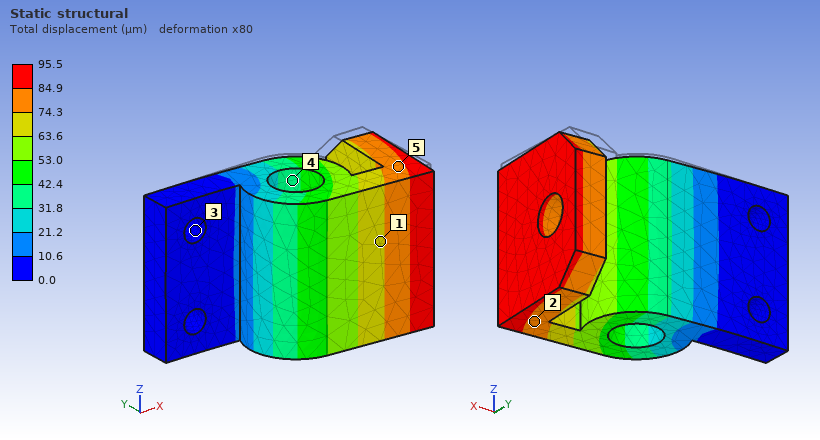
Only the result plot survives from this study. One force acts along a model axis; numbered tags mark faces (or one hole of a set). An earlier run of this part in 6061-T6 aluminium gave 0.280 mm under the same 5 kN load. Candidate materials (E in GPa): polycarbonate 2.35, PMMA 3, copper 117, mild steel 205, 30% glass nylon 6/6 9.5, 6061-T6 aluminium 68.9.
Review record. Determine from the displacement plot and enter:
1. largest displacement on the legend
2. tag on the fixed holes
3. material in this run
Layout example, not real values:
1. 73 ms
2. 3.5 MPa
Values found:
1. 95.5 µm
2. 3
3. mild steel
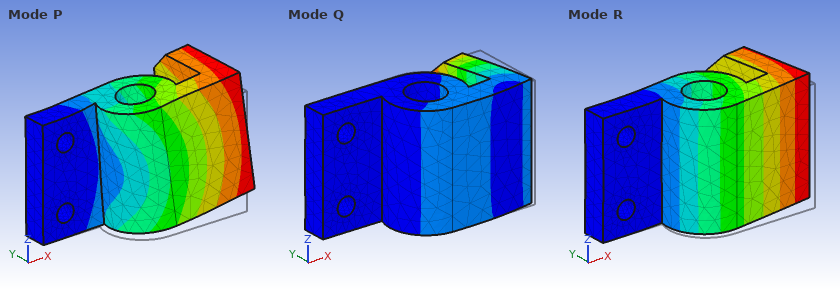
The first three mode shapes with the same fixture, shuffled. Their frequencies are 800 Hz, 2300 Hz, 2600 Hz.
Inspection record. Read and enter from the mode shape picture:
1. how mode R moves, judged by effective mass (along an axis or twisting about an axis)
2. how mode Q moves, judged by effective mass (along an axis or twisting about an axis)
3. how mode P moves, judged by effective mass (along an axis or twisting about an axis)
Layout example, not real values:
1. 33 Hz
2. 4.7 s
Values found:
1. along Y
2. along X
3. along Z
